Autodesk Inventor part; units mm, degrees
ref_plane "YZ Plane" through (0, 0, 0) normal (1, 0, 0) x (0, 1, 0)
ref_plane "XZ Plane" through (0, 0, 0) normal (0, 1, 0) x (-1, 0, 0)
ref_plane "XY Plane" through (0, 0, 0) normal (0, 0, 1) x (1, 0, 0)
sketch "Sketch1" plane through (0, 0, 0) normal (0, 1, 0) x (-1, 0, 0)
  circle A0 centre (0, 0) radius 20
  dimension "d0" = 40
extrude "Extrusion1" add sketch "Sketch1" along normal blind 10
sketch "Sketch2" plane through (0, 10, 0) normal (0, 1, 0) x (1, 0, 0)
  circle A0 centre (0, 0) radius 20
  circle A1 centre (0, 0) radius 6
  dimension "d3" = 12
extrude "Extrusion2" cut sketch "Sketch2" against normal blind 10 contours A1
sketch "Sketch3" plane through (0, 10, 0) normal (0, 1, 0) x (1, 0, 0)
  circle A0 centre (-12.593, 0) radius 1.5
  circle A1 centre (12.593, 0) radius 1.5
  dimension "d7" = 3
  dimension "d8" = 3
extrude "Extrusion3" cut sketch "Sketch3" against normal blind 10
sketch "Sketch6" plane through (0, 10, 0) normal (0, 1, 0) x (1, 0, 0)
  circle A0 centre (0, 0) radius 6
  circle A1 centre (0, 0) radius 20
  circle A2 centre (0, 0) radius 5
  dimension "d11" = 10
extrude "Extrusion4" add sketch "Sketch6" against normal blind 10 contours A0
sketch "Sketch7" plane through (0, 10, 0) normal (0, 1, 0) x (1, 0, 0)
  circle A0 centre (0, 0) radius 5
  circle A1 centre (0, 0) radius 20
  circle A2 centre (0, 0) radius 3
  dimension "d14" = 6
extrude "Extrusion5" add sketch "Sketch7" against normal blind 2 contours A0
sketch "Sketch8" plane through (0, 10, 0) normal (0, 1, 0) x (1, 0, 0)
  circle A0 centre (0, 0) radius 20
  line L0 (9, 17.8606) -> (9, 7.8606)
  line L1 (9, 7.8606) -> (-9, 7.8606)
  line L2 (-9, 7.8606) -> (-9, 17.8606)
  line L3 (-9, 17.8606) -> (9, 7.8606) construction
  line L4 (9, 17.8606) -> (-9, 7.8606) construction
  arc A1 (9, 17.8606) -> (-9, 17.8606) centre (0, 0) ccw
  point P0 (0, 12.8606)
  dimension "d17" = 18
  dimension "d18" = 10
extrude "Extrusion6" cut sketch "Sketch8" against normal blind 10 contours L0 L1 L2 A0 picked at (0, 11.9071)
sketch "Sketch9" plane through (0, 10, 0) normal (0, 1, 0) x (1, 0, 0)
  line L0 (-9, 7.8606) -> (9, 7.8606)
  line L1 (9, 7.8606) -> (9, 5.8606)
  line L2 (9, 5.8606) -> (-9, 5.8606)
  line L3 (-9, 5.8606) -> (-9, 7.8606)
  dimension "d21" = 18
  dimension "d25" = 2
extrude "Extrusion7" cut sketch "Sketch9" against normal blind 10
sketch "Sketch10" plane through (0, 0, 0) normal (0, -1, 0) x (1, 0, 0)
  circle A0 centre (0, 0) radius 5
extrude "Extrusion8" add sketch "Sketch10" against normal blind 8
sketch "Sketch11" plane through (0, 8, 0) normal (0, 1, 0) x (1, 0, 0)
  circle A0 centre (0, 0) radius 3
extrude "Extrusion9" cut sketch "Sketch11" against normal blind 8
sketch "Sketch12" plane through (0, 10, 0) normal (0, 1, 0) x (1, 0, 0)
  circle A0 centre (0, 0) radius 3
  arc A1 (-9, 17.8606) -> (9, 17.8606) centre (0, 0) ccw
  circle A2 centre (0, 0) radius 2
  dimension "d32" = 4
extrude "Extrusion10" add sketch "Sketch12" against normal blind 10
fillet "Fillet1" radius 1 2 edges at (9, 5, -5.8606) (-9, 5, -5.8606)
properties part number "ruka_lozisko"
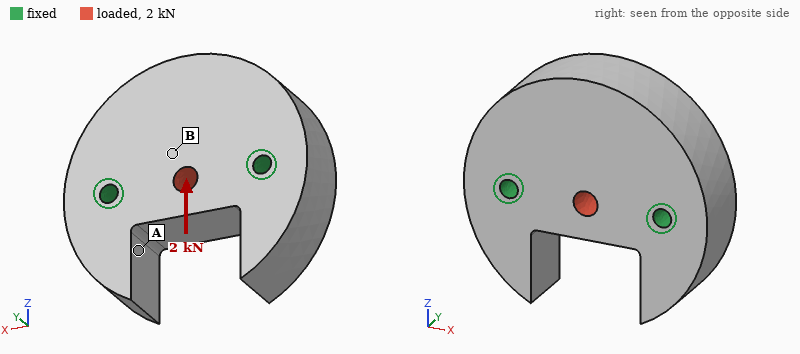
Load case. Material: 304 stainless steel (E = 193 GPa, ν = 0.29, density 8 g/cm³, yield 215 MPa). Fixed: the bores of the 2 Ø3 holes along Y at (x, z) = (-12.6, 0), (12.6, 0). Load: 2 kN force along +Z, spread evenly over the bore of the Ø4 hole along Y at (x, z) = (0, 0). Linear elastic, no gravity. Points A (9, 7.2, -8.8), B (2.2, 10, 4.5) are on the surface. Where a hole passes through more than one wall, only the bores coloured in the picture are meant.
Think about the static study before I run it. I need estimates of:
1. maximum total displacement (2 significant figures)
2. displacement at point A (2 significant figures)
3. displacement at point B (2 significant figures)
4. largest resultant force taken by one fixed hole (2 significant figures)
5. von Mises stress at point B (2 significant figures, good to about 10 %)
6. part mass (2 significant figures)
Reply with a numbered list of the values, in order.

1. 1.6 µm
2. 0.57 µm
3. 0.98 µm
4. 1.0 kN
5. 13 MPa
6. 79 g
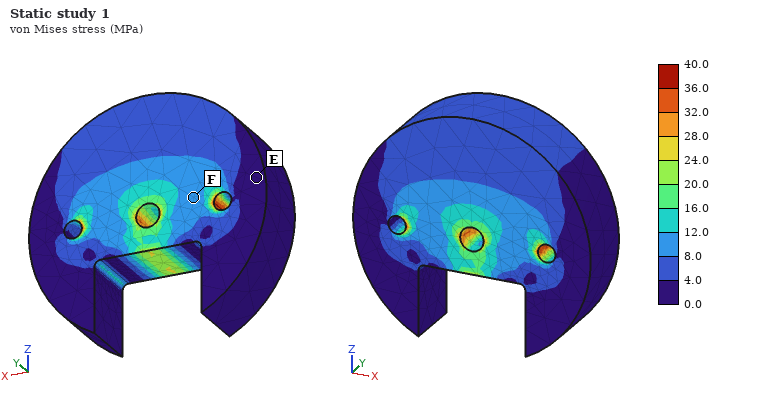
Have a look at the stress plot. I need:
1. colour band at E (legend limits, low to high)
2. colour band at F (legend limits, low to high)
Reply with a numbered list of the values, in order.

1. 0.0 to 4.0 MPa
2. 8.0 to 12.0 MPa
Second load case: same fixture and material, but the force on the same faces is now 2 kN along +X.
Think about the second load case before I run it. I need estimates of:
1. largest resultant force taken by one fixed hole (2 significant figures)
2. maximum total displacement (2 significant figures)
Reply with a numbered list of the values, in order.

1. 1.0 kN
2. 0.72 µm
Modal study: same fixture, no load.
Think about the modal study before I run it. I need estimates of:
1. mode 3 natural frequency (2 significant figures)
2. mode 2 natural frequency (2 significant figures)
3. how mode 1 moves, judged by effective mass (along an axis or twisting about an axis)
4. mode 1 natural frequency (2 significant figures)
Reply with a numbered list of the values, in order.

1. 30 kHz
2. 30 kHz
3. along Y
4. 16 kHz
